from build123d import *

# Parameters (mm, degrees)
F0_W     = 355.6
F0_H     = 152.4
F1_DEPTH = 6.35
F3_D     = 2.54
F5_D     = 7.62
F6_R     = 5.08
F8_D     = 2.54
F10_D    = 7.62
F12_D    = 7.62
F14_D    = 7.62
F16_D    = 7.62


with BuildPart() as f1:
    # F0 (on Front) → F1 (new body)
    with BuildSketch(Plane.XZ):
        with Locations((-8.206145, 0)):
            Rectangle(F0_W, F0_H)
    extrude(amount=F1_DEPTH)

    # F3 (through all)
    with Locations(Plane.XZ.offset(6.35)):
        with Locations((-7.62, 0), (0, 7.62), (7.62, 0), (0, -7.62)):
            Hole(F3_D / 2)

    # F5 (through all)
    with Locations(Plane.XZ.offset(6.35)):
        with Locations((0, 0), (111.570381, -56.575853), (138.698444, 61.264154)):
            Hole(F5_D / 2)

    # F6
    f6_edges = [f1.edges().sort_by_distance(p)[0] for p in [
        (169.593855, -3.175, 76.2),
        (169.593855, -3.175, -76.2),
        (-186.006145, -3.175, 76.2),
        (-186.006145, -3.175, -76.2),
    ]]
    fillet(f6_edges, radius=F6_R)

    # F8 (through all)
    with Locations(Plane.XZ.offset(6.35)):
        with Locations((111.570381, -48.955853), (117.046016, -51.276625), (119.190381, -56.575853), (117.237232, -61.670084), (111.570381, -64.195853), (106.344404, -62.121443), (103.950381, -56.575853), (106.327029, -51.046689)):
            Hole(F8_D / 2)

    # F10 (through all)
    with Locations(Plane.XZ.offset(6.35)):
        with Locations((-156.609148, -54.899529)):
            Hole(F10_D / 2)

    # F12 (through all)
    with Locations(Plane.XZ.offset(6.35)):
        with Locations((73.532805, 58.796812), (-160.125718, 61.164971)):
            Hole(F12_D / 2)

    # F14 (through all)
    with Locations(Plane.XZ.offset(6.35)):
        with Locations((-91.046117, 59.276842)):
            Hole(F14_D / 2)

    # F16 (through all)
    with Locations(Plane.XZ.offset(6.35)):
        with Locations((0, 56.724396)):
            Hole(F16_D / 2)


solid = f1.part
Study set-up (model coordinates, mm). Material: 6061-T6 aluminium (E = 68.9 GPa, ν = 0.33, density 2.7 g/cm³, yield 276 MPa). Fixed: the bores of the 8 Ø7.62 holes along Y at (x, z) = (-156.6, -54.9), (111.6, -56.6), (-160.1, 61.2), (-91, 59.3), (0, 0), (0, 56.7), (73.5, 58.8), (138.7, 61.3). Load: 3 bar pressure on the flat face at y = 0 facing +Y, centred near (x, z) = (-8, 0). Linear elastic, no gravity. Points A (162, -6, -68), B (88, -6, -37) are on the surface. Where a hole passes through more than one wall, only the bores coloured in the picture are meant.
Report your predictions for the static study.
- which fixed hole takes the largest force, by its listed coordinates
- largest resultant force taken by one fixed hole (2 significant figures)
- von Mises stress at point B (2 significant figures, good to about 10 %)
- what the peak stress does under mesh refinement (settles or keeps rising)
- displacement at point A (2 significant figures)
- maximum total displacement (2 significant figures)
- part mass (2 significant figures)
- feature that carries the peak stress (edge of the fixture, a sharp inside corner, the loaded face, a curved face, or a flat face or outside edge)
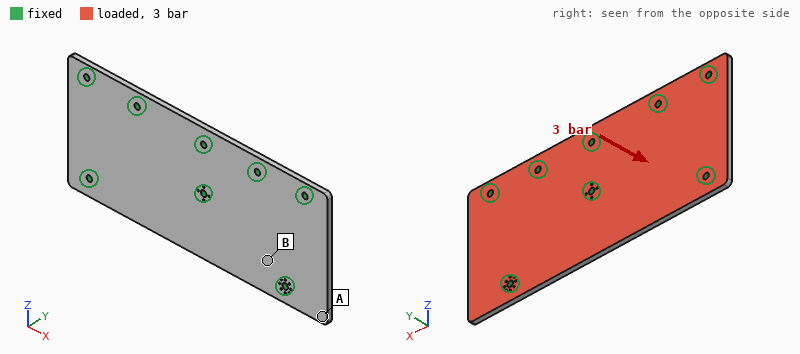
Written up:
(0, 0)
4.2 kN
43 MPa
keeps rising
0.21 mm
0.88 mm
920 g
a sharp inside corner
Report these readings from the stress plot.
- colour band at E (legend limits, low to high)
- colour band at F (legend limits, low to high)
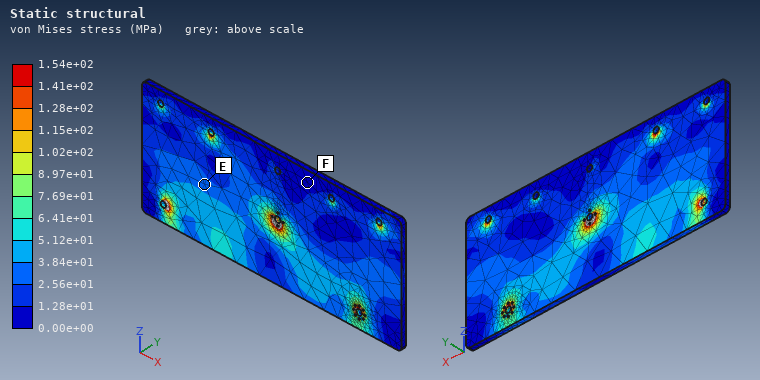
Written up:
2.56e+01 to 3.84e+01 MPa
0.00e+00 to 1.28e+01 MPa
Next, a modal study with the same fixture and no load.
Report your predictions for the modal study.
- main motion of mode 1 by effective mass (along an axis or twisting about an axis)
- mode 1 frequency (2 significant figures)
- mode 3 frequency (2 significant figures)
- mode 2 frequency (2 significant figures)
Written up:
along Y
950 Hz
1500 Hz
1400 Hz
